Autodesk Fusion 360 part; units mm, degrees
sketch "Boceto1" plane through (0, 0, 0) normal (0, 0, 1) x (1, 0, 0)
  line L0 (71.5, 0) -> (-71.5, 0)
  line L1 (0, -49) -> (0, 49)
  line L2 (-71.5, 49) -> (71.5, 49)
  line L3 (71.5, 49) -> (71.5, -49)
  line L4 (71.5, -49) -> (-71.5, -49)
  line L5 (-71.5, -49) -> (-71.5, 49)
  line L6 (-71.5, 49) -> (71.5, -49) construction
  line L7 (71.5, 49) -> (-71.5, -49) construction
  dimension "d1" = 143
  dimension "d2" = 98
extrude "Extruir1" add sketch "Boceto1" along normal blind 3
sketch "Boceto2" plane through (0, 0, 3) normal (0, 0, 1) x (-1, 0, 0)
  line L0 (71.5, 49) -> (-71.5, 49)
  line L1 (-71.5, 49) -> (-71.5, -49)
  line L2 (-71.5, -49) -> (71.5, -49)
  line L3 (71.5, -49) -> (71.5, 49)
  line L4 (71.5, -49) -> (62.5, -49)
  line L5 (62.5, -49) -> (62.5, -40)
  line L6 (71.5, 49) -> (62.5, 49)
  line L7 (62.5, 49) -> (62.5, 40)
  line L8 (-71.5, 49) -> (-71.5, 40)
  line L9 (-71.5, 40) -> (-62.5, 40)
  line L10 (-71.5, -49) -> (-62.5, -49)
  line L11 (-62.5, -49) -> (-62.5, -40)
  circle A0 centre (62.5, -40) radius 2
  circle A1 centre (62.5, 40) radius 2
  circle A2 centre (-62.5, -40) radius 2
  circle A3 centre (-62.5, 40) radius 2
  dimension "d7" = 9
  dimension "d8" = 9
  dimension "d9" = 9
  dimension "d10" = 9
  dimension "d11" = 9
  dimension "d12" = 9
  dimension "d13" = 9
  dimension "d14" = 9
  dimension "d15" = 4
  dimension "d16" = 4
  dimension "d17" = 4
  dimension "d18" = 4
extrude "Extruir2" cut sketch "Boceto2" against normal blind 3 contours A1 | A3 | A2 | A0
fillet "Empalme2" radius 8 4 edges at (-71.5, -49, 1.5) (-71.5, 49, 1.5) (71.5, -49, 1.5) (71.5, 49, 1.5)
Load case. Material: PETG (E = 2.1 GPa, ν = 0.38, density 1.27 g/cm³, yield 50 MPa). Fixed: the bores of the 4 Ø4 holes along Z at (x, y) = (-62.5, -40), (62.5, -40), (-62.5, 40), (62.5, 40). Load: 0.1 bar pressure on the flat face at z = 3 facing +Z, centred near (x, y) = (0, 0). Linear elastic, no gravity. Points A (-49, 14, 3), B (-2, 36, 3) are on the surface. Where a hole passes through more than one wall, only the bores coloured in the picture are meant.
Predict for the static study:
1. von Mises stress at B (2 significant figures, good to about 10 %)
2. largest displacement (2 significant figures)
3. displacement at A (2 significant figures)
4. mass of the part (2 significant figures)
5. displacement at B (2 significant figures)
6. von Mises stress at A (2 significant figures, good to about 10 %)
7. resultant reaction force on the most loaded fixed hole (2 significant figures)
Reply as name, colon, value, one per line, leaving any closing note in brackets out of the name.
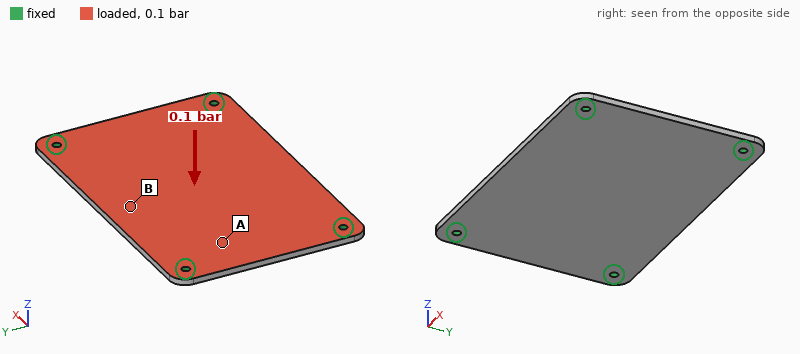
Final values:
von Mises stress at B: 5.1 MPa
largest displacement: 2.0 mm
displacement at A: 0.68 mm
mass of the part: 53 g
displacement at B: 1.8 mm
von Mises stress at A: 2.2 MPa
resultant reaction force on the most loaded fixed hole: 35 N
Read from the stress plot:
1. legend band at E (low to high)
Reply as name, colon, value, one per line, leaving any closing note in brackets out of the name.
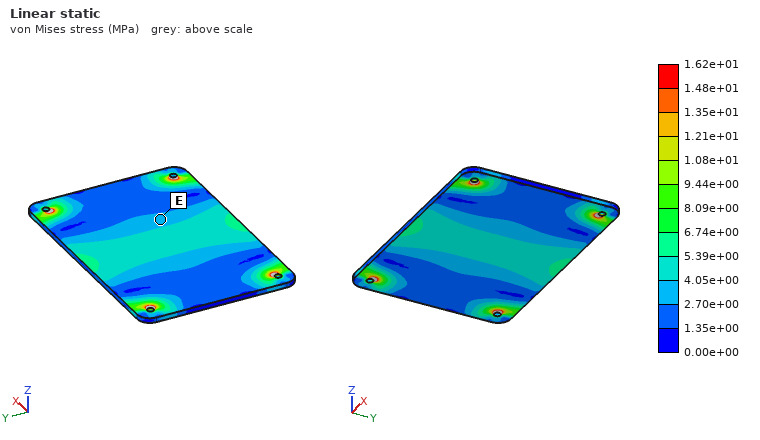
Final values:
legend band at E: 2.70e+00 to 4.05e+00 MPa
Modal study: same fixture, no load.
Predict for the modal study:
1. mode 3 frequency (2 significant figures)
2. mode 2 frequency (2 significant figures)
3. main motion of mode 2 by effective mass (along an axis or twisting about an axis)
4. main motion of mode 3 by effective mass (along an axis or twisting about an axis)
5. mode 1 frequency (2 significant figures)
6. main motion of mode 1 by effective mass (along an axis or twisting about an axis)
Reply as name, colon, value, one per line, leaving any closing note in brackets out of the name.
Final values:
mode 3 frequency: 530 Hz
mode 2 frequency: 330 Hz
main motion of mode 2 by effective mass: twisting about X
main motion of mode 3 by effective mass: twisting about Y
mode 1 frequency: 210 Hz
main motion of mode 1 by effective mass: along Z
